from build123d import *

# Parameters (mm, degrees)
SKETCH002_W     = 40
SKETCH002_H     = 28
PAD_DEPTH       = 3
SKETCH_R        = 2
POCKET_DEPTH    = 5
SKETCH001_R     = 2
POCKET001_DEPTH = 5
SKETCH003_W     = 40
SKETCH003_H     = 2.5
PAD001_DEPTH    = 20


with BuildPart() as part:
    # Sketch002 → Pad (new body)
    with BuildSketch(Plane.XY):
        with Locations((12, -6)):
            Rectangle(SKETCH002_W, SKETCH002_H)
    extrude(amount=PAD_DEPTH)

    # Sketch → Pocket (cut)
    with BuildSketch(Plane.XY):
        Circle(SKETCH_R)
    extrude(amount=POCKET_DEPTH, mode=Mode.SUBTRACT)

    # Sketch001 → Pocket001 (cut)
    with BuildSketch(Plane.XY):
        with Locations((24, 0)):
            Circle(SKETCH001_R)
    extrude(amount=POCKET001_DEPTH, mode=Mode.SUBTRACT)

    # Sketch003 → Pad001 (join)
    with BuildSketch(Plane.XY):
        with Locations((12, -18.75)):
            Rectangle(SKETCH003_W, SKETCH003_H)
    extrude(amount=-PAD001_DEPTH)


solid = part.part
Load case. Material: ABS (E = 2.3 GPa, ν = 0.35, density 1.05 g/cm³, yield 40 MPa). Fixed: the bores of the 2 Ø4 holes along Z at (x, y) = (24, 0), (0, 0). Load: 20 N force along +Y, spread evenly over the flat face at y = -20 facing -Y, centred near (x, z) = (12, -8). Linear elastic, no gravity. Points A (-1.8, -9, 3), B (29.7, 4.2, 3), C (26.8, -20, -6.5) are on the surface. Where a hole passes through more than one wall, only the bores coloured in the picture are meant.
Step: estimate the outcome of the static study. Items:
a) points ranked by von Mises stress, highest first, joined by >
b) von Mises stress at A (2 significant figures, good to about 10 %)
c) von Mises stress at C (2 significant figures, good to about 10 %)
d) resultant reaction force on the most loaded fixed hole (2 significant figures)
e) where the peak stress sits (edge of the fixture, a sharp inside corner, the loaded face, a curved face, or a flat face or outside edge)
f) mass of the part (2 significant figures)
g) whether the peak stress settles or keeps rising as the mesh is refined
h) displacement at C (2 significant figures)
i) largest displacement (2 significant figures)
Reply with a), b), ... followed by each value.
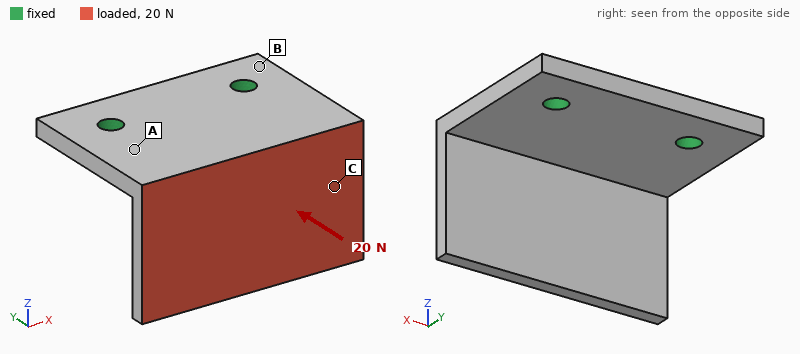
a) A > C > B
b) 2.9 MPa
c) 1.7 MPa
d) 10 N
e) edge of the fixture
f) 5.5 g
g) keeps rising
h) 0.25 mm
i) 0.54 mm
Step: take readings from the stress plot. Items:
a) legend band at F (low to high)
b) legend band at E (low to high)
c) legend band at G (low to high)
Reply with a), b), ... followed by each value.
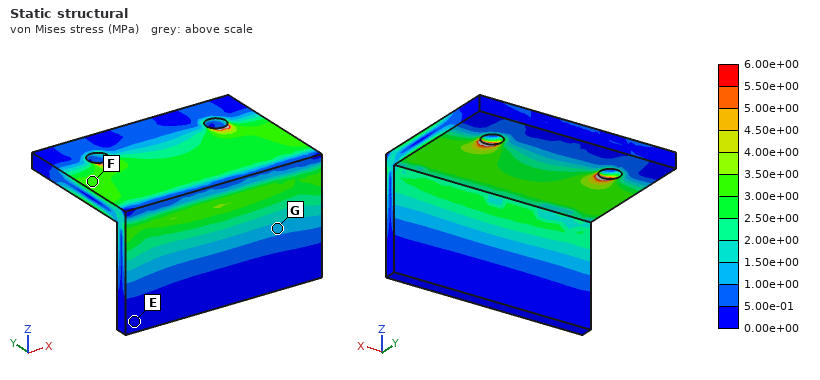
a) 3.00e+00 to 3.50e+00 MPa
b) 0.00e+00 to 5.00e-01 MPa
c) 1.00e+00 to 1.50e+00 MPa
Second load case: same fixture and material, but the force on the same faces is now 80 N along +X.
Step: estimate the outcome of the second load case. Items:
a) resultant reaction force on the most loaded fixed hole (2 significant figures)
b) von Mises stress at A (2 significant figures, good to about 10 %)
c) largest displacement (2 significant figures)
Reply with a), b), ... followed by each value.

a) 77 N
b) 5.1 MPa
c) 0.61 mm
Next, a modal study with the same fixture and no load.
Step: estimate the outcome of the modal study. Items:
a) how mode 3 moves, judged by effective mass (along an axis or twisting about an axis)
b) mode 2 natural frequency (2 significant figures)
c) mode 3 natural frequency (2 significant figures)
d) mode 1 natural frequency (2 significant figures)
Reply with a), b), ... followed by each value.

a) along Z
b) 1100 Hz
c) 1600 Hz
d) 650 Hz
